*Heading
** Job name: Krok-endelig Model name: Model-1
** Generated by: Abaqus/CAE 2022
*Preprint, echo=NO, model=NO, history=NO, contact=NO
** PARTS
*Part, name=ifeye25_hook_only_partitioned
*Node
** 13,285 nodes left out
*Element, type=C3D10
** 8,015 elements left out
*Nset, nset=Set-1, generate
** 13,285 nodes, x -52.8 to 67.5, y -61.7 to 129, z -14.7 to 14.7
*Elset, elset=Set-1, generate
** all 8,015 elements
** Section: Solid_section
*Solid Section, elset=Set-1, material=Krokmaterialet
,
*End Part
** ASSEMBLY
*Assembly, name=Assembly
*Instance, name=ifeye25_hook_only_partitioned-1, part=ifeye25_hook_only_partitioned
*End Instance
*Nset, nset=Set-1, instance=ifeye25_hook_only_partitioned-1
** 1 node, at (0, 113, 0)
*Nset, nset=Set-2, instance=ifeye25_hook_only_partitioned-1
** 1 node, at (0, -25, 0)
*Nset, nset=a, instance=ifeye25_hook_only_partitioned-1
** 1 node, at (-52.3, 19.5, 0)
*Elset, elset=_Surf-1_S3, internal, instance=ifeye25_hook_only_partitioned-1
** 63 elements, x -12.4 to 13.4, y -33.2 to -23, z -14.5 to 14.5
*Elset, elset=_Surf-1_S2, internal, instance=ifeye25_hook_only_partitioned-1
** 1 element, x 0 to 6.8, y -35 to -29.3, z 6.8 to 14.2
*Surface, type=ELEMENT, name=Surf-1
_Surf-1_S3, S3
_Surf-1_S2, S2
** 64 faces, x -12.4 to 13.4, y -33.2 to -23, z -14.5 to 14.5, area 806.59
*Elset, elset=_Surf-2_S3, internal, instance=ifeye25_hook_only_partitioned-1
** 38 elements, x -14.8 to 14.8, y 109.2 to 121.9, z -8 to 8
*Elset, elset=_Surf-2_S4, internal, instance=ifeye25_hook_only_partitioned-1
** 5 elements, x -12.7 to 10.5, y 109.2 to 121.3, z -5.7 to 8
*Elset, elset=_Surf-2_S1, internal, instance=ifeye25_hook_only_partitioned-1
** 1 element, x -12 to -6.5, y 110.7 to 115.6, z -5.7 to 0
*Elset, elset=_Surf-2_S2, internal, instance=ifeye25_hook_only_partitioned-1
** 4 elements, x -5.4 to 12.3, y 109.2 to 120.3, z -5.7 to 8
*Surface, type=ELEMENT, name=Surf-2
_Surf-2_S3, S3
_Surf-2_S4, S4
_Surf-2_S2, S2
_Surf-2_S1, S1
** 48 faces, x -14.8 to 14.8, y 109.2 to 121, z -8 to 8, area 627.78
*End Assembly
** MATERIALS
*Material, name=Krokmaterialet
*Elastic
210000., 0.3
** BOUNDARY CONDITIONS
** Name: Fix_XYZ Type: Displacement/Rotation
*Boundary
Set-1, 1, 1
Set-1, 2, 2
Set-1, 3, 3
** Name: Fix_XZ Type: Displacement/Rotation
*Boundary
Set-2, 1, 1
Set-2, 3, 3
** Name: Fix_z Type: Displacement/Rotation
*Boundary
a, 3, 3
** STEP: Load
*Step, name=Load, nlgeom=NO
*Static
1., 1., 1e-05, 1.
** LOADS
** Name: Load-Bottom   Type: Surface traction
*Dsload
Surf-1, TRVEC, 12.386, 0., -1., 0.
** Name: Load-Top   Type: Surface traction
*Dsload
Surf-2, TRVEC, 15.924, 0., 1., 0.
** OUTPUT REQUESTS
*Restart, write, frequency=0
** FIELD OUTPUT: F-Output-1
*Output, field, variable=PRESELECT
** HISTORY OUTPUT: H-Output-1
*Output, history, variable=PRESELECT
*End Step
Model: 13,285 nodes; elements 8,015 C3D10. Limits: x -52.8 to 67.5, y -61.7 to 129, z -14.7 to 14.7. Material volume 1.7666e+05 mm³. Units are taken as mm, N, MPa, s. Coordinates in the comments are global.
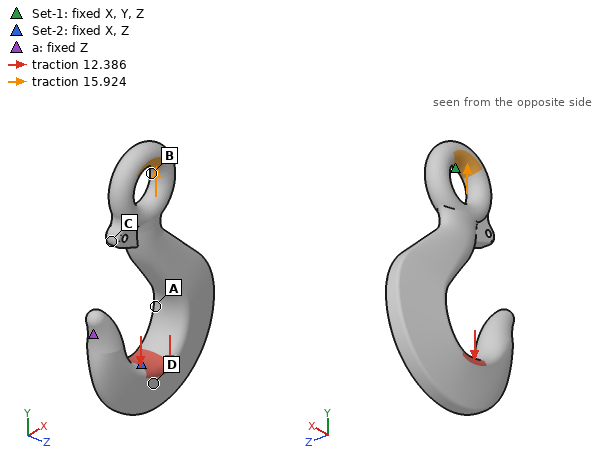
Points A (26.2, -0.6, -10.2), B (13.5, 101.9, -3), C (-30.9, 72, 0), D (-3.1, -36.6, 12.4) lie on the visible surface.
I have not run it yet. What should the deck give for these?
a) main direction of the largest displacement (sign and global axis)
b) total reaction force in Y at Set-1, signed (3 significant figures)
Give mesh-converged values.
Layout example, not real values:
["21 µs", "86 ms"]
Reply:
["-Y", "-6.44 N"]
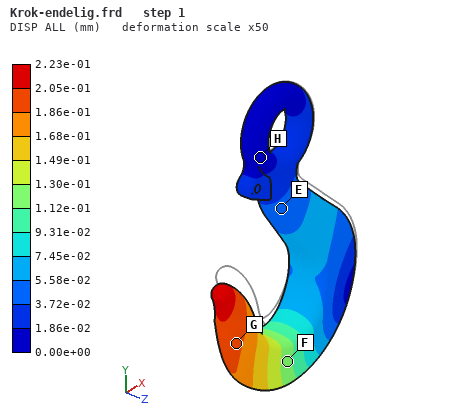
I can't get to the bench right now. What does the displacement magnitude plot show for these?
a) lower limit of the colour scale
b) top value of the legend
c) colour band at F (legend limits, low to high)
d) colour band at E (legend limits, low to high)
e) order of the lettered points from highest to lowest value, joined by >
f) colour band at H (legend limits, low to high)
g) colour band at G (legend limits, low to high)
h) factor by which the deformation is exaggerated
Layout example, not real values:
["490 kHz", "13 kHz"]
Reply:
["0.00e+00 mm", "2.23e-01 mm", "1.12e-01 to 1.30e-01 mm", "3.72e-02 to 5.58e-02 mm", "G > F > E > H", "0.00e+00 to 1.86e-02 mm", "1.86e-01 to 2.05e-01 mm", "50"]
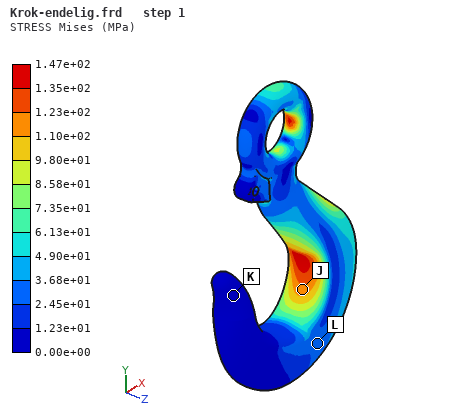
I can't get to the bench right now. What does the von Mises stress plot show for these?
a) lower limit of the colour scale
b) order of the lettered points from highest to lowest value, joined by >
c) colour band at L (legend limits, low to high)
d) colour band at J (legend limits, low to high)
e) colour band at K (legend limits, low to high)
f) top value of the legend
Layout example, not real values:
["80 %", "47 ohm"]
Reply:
["0.00e+00 MPa", "J > L > K", "2.45e+01 to 3.68e+01 MPa", "1.10e+02 to 1.23e+02 MPa", "0.00e+00 to 1.23e+01 MPa", "1.47e+02 MPa"]
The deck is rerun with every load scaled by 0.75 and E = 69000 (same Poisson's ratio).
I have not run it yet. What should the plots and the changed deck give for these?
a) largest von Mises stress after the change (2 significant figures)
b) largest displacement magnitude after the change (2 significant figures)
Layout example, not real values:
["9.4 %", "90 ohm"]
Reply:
["110 MPa", "0.51 mm"]
